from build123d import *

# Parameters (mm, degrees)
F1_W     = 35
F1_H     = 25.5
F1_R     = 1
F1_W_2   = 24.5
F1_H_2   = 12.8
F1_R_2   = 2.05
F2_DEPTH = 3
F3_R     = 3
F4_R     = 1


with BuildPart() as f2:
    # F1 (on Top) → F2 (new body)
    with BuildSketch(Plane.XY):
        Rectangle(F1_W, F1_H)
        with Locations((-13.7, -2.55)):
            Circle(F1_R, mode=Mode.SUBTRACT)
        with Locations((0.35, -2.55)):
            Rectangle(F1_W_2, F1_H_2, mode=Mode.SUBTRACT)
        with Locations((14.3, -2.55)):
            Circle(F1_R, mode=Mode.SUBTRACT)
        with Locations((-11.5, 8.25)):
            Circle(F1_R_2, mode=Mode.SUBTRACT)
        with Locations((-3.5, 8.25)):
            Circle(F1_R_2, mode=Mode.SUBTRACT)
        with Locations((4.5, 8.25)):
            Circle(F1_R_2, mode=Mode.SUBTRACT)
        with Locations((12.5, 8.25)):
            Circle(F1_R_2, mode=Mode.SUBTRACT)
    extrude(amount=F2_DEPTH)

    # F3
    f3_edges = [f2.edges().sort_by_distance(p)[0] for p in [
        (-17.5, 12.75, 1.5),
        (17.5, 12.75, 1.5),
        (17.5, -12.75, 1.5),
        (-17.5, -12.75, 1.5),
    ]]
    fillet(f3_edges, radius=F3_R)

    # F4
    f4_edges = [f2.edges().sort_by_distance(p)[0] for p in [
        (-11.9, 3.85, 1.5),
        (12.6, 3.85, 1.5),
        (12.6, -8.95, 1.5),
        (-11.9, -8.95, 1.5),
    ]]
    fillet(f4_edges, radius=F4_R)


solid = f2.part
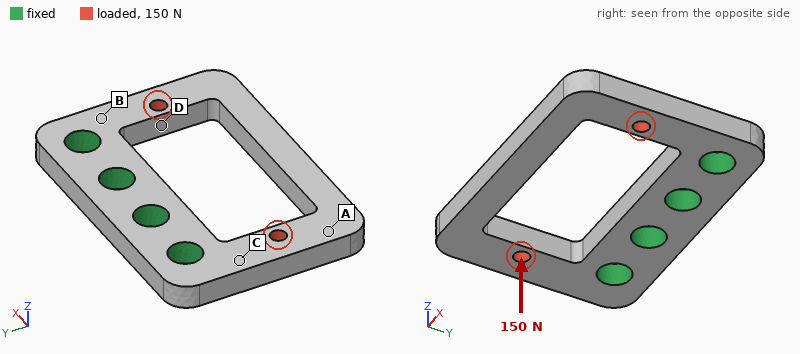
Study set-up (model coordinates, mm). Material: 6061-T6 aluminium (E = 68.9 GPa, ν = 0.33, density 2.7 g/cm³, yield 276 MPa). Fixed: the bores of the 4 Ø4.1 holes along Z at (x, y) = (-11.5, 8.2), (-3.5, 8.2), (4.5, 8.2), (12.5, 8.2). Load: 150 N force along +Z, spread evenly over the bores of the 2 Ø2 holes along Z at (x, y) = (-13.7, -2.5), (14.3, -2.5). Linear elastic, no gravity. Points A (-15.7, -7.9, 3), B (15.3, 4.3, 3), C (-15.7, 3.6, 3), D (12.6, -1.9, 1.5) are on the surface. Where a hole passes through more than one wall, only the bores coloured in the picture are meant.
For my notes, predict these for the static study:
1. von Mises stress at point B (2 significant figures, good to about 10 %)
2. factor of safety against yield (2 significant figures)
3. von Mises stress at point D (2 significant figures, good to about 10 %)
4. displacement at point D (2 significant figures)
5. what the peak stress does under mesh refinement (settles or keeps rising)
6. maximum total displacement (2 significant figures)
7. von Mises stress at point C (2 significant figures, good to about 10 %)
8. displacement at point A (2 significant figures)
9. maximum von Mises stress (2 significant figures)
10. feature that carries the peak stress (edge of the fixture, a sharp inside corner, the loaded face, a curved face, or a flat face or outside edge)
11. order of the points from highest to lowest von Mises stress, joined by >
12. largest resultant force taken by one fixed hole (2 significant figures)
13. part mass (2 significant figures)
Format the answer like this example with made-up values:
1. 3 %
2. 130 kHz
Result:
1. 55 MPa
2. 2.5
3. 22 MPa
4. 24 µm
5. settles
6. 68 µm
7. 44 MPa
8. 46 µm
9. 110 MPa
10. a curved face
11. B > C > D > A
12. 81 N
13. 4.2 g
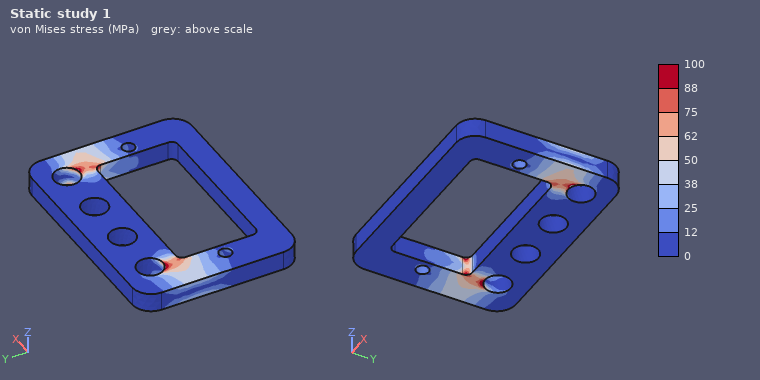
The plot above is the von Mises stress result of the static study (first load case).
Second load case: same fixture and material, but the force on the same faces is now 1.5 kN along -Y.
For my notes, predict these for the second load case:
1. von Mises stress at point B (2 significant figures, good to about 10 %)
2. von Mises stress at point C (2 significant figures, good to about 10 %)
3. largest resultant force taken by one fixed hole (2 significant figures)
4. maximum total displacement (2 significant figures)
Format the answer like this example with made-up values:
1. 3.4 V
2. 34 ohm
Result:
1. 49 MPa
2. 34 MPa
3. 790 N
4. 13 µm
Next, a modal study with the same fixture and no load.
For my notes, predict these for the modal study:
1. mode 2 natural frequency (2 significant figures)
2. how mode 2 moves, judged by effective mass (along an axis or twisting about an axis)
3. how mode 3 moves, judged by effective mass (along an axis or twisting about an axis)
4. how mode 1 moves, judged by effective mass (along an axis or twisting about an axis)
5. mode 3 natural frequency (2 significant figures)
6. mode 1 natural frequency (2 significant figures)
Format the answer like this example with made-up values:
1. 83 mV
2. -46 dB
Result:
1. 7200 Hz
2. twisting about Y
3. along X
4. along Z
5. 9600 Hz
6. 4000 Hz
